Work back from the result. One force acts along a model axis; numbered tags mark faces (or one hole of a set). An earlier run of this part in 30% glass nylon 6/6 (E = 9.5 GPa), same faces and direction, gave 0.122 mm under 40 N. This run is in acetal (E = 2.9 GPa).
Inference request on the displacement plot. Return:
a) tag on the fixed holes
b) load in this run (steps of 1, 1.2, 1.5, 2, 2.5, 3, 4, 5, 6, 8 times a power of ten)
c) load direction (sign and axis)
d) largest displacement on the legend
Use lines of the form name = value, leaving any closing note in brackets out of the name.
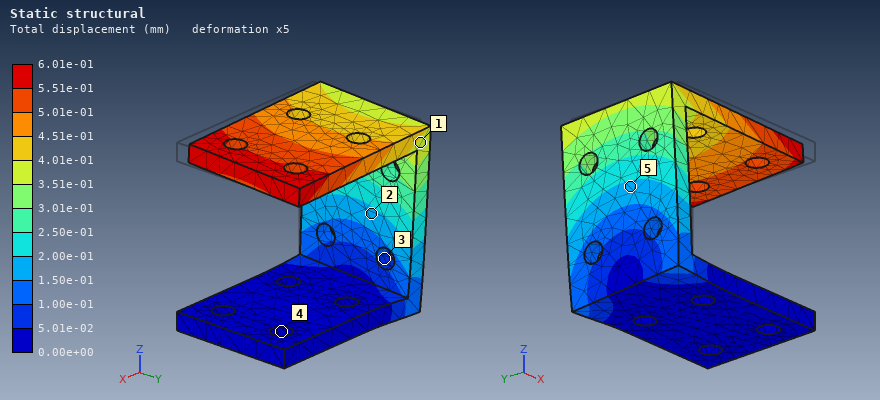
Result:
tag on the fixed holes = 4
load in this run = 60 N
load direction = +Y
largest displacement on the legend = 6.01e-01 mm
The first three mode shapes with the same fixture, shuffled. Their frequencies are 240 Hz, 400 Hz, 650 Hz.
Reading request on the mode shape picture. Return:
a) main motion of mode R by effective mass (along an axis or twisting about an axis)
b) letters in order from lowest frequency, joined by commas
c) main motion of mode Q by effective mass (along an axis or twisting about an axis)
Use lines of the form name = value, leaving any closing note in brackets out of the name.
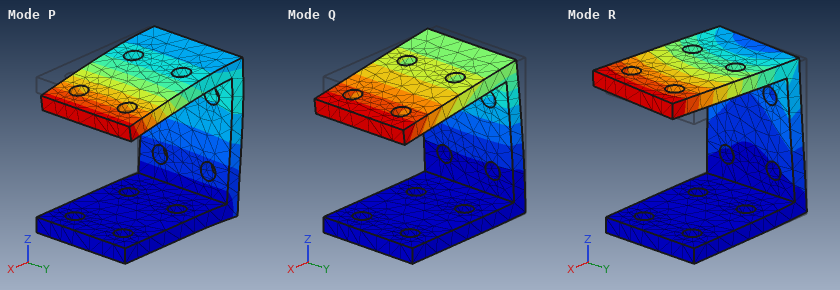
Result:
main motion of mode R by effective mass = along Y
letters in order from lowest frequency, joined by commas = Q, R, P
main motion of mode Q by effective mass = along X
